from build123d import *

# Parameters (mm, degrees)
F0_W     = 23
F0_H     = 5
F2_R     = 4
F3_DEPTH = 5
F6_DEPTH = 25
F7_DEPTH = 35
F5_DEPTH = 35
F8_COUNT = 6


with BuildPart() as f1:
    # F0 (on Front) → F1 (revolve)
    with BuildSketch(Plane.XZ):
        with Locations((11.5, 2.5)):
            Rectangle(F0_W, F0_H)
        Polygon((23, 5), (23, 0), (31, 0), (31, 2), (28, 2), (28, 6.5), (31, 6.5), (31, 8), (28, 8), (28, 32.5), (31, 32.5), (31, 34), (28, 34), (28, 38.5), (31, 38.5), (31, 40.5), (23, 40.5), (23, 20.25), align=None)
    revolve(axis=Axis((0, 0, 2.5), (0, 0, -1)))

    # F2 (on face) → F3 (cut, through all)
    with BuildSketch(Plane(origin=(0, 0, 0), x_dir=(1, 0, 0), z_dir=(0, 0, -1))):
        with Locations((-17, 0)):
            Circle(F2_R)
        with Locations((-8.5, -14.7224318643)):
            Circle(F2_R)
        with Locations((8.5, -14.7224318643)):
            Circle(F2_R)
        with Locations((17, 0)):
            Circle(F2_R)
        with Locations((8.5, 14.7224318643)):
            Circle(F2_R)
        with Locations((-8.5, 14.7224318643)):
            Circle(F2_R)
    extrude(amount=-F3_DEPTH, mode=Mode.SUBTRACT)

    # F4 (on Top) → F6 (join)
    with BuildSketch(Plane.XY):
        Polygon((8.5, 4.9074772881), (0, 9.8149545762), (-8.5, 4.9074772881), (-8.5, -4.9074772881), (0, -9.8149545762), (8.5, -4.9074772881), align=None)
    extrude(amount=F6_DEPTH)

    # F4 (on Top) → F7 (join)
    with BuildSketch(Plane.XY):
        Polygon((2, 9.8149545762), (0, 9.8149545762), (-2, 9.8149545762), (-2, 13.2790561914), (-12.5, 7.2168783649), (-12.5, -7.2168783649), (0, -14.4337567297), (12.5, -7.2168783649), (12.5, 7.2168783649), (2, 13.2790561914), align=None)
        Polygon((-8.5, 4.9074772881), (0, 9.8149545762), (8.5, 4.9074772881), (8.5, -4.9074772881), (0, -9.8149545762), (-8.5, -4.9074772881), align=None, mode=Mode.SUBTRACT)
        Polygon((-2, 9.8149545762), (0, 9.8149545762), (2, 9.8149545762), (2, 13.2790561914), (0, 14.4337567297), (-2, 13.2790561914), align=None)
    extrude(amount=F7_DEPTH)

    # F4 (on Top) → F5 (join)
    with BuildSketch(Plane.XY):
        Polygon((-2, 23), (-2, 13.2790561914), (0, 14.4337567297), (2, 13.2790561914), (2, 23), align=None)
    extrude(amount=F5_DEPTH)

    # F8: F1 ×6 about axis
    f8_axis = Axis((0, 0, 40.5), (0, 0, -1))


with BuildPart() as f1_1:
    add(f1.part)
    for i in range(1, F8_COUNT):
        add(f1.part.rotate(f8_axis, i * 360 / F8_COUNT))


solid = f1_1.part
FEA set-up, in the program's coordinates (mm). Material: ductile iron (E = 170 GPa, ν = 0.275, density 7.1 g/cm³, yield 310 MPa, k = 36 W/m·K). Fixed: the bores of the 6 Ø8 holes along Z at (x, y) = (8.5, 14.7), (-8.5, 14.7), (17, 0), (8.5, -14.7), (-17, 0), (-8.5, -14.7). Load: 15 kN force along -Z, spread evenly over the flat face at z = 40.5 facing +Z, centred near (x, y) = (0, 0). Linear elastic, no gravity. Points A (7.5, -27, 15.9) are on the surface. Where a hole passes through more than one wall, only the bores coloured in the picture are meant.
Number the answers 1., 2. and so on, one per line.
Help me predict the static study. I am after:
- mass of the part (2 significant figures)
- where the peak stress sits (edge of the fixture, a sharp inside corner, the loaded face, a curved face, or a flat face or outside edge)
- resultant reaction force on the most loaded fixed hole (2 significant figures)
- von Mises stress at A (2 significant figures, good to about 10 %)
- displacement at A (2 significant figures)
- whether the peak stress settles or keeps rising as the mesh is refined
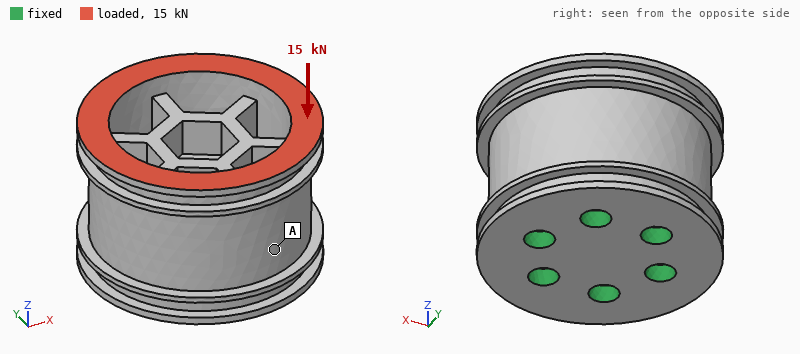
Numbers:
1. 450 g
2. edge of the fixture
3. 2.5 kN
4. 12 MPa
5. 3.0 µm
6. keeps rising
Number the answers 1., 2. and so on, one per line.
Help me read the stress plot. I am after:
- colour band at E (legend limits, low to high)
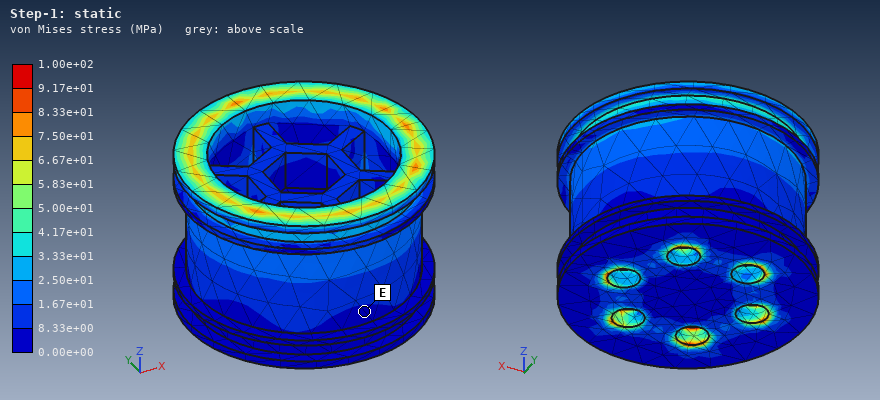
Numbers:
1. 0.00e+00 to 8.33e+00 MPa
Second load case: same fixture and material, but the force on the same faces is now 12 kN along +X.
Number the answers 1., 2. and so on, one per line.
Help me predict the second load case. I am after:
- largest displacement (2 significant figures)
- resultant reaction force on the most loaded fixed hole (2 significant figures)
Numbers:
1. 40 µm
2. 7.8 kN
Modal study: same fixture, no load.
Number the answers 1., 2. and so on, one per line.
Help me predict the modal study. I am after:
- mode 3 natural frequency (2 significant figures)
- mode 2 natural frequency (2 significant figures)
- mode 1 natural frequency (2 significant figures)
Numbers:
1. 15 kHz
2. 9500 Hz
3. 9500 Hz
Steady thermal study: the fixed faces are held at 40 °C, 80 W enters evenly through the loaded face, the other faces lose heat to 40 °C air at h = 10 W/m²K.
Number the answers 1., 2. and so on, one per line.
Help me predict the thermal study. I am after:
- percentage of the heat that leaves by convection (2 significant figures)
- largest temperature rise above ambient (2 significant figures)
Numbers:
1. 10.0 %
2. 85 K
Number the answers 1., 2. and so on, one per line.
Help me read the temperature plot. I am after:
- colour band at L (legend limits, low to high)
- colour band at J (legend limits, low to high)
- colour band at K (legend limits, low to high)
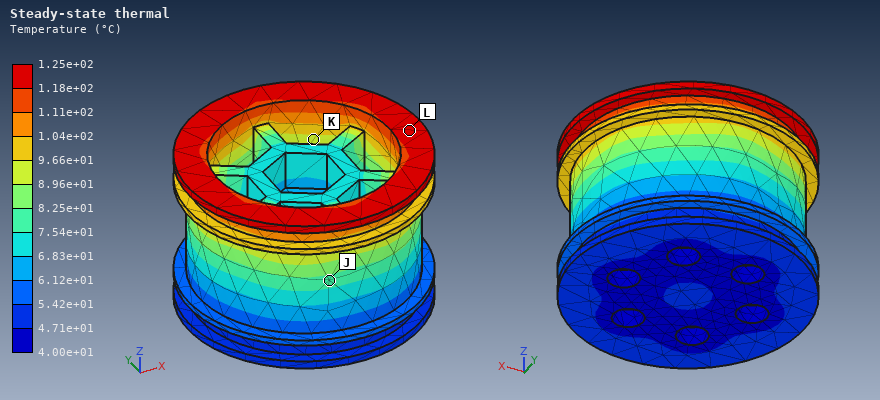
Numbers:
1. 1.18e+02 to 1.25e+02 °C
2. 7.54e+01 to 8.25e+01 °C
3. 8.96e+01 to 9.66e+01 °C
